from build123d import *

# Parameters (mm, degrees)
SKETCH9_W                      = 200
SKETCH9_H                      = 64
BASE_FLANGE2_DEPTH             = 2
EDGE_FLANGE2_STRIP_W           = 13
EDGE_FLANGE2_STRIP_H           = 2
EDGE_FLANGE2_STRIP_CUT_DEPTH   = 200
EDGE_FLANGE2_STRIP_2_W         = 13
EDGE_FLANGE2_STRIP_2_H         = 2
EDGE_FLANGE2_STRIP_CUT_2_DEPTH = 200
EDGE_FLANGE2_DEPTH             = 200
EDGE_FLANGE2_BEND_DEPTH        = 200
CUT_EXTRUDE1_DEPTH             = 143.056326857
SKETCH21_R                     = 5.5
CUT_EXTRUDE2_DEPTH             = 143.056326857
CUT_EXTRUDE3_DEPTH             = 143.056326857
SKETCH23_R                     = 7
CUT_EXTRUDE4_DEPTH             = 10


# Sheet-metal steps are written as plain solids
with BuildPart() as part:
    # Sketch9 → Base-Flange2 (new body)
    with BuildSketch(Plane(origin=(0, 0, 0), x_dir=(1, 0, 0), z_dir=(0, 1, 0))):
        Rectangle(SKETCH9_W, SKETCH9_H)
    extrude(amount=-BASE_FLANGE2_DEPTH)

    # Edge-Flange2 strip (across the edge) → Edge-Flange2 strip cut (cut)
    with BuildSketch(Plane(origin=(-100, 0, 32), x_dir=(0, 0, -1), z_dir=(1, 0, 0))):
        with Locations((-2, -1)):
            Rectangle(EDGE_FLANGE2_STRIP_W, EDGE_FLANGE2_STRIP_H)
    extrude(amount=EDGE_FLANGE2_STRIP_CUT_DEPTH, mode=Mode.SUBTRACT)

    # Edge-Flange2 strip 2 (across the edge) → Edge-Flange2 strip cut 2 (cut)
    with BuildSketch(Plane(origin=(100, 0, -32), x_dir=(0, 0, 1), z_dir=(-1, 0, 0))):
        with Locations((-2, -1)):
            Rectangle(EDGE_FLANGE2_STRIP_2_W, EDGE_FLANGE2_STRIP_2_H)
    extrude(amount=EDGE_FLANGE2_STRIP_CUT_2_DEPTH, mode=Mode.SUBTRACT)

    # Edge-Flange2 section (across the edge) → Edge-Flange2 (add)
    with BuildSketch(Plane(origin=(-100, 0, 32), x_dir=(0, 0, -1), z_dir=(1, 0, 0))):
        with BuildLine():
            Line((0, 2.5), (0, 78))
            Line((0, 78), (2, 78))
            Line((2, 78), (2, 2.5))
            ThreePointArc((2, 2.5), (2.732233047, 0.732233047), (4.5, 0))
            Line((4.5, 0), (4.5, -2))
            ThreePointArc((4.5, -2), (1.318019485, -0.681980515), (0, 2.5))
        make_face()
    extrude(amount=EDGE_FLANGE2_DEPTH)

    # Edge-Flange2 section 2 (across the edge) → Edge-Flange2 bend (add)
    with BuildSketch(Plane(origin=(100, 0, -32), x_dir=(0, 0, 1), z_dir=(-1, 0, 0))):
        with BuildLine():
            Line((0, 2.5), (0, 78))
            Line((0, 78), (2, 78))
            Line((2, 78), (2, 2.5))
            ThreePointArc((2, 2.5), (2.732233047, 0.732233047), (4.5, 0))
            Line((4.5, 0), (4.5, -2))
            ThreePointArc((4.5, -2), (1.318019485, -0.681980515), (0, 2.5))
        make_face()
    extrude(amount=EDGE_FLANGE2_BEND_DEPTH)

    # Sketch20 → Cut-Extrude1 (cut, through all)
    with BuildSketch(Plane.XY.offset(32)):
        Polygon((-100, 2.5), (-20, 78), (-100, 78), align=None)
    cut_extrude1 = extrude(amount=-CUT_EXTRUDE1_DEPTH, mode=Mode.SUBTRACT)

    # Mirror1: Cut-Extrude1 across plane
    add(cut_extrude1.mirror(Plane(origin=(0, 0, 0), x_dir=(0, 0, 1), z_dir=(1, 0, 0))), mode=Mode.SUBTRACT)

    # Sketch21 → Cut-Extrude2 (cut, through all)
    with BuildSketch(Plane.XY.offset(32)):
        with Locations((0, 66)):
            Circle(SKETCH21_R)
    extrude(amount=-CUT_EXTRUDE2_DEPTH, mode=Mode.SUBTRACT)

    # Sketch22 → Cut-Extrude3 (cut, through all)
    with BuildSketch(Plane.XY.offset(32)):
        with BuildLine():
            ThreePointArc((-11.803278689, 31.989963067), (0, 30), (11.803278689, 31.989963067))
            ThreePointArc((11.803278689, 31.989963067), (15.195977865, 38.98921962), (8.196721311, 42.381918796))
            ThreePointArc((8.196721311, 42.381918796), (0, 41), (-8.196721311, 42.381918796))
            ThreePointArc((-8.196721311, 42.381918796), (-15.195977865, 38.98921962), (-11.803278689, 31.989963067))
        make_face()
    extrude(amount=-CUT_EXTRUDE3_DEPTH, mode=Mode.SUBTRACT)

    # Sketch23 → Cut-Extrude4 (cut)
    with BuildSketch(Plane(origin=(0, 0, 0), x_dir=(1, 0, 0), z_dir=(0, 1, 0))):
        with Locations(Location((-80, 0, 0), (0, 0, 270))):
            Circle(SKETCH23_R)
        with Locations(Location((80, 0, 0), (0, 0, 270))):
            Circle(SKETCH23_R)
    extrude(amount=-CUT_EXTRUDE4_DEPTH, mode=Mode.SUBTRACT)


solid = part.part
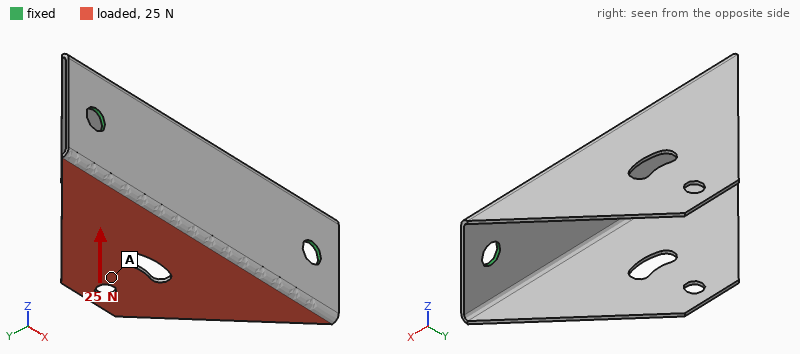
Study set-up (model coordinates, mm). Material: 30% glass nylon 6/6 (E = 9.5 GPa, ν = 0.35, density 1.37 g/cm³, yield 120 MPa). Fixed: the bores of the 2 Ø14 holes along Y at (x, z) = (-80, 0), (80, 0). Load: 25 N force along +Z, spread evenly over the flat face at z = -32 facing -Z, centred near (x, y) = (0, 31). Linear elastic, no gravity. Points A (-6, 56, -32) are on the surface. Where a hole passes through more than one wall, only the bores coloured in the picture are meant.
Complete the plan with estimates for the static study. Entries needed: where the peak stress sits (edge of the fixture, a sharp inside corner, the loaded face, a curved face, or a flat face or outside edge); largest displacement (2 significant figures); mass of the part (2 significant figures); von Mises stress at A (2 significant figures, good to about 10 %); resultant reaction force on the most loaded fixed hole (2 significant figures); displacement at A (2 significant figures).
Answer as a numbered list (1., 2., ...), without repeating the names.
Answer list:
1. a flat face or outside edge
2. 2.6 mm
3. 83 g
4. 1.3 MPa
5. 13 N
6. 1.8 mm
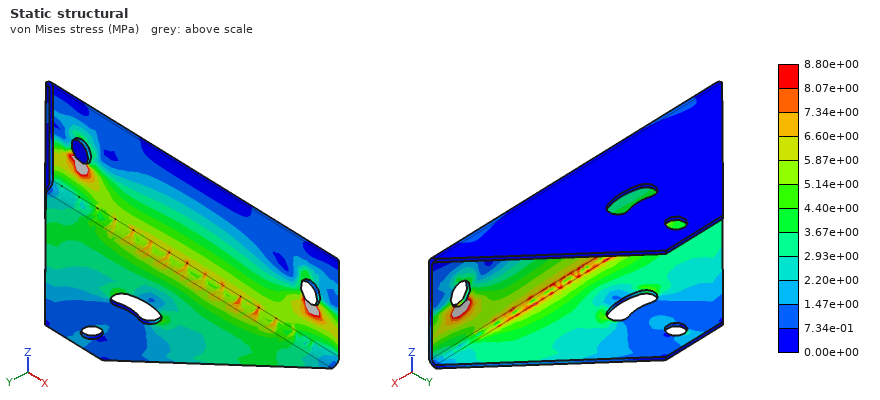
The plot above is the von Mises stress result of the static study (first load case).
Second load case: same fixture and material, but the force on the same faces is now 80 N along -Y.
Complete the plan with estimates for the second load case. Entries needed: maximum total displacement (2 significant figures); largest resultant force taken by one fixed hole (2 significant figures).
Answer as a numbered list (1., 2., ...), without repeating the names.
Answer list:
1. 2.3 mm
2. 45 N
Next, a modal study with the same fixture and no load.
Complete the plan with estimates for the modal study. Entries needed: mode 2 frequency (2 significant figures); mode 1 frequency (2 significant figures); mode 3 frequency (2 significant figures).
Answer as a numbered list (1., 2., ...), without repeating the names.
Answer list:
1. 140 Hz
2. 130 Hz
3. 330 Hz
